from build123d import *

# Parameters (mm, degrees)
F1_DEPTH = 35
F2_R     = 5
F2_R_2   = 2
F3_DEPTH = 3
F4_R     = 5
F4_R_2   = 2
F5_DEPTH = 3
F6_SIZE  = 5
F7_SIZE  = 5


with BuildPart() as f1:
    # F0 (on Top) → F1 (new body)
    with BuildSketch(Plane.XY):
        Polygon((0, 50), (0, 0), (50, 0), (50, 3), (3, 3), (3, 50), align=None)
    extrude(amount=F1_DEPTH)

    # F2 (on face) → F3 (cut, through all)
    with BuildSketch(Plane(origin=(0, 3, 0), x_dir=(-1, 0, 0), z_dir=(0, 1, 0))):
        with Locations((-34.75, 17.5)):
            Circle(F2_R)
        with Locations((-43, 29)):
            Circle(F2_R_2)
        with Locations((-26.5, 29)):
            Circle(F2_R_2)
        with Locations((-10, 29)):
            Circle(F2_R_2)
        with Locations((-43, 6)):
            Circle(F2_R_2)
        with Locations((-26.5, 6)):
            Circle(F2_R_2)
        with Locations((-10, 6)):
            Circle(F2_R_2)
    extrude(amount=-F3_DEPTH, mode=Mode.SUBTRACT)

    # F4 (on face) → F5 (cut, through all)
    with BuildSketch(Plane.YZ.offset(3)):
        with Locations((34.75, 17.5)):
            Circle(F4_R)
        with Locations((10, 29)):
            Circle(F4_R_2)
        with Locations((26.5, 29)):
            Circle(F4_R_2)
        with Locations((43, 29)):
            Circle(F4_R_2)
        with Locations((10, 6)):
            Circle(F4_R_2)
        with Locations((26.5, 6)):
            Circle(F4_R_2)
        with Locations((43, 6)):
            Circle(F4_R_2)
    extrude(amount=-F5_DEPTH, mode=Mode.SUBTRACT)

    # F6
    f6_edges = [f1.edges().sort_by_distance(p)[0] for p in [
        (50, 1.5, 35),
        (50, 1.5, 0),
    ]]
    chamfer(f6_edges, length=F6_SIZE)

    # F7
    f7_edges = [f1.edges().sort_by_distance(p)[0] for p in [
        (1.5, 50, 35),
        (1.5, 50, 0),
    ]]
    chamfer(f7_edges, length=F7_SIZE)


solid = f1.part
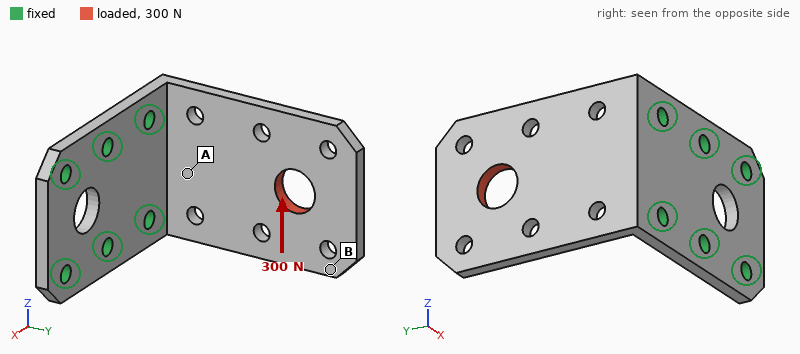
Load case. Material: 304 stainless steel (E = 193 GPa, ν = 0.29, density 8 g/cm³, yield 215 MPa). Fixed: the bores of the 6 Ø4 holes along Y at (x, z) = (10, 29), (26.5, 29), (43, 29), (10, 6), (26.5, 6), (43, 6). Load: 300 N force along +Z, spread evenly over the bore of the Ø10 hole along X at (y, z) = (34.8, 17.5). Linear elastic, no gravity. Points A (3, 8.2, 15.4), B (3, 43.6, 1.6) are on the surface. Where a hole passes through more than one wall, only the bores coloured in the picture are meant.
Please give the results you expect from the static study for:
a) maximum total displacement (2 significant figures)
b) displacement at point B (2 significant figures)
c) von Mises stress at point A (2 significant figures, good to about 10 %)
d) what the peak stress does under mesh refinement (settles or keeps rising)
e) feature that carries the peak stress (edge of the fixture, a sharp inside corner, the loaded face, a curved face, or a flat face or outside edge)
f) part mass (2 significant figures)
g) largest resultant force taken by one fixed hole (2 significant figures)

37 µm
34 µm
23 MPa
keeps rising
edge of the fixture
73 g
450 N
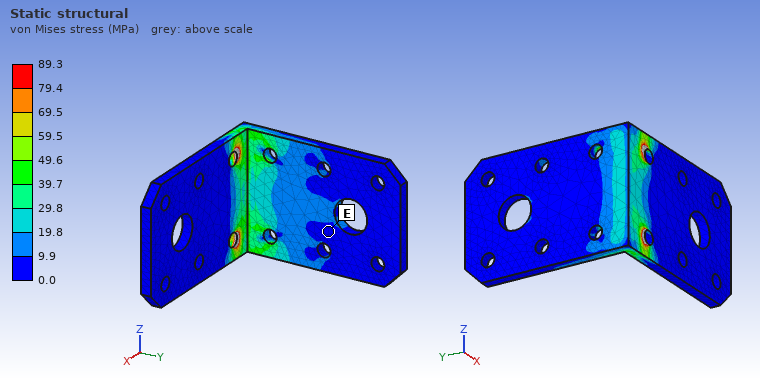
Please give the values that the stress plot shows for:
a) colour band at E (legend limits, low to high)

0.0 to 9.9 MPa
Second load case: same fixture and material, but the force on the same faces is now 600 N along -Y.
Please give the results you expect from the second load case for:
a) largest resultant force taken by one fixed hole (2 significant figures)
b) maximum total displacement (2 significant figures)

330 N
63 µm
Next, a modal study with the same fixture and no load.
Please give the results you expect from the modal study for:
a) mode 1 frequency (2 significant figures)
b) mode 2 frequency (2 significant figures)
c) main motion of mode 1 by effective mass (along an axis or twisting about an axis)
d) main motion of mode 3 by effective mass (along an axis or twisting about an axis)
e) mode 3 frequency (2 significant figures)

860 Hz
2800 Hz
along X
along Z
3800 Hz
